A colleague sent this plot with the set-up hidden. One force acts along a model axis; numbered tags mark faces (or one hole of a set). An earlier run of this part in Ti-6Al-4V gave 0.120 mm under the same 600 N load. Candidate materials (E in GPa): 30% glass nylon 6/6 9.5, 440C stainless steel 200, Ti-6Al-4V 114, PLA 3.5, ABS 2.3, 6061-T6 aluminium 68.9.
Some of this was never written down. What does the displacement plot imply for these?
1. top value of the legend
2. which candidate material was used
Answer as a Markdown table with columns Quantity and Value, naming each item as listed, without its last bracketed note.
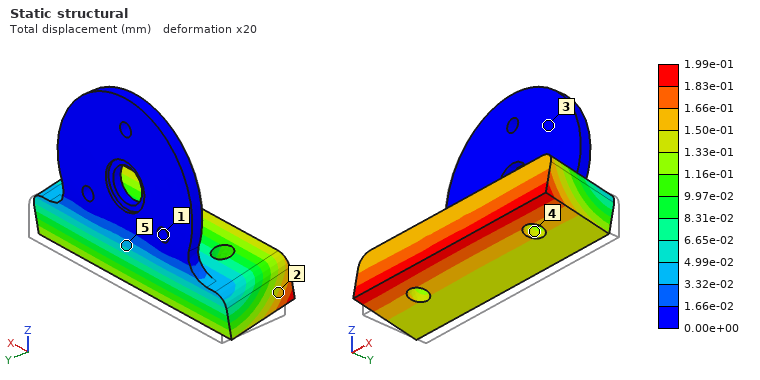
| Quantity | Value |
|---|---|
| top value of the legend | 1.99e-01 mm |
| which candidate material was used | 6061-T6 aluminium |
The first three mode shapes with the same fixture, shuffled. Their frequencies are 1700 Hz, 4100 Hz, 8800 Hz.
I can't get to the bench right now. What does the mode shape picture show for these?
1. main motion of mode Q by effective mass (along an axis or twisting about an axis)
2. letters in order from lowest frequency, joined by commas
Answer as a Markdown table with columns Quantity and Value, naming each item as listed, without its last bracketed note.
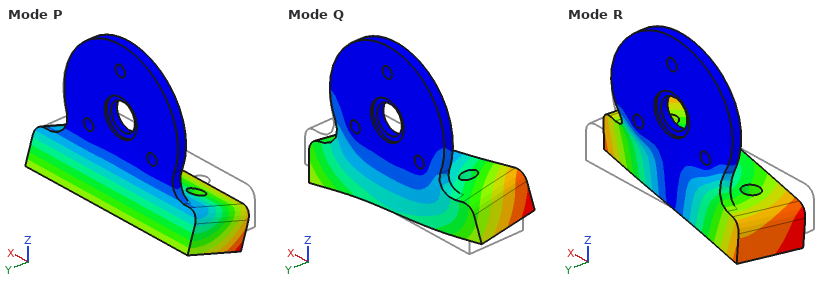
| Quantity | Value |
|---|---|
| main motion of mode Q by effective mass | along X |
| letters in order from lowest frequency, joined by commas | P, R, Q |
